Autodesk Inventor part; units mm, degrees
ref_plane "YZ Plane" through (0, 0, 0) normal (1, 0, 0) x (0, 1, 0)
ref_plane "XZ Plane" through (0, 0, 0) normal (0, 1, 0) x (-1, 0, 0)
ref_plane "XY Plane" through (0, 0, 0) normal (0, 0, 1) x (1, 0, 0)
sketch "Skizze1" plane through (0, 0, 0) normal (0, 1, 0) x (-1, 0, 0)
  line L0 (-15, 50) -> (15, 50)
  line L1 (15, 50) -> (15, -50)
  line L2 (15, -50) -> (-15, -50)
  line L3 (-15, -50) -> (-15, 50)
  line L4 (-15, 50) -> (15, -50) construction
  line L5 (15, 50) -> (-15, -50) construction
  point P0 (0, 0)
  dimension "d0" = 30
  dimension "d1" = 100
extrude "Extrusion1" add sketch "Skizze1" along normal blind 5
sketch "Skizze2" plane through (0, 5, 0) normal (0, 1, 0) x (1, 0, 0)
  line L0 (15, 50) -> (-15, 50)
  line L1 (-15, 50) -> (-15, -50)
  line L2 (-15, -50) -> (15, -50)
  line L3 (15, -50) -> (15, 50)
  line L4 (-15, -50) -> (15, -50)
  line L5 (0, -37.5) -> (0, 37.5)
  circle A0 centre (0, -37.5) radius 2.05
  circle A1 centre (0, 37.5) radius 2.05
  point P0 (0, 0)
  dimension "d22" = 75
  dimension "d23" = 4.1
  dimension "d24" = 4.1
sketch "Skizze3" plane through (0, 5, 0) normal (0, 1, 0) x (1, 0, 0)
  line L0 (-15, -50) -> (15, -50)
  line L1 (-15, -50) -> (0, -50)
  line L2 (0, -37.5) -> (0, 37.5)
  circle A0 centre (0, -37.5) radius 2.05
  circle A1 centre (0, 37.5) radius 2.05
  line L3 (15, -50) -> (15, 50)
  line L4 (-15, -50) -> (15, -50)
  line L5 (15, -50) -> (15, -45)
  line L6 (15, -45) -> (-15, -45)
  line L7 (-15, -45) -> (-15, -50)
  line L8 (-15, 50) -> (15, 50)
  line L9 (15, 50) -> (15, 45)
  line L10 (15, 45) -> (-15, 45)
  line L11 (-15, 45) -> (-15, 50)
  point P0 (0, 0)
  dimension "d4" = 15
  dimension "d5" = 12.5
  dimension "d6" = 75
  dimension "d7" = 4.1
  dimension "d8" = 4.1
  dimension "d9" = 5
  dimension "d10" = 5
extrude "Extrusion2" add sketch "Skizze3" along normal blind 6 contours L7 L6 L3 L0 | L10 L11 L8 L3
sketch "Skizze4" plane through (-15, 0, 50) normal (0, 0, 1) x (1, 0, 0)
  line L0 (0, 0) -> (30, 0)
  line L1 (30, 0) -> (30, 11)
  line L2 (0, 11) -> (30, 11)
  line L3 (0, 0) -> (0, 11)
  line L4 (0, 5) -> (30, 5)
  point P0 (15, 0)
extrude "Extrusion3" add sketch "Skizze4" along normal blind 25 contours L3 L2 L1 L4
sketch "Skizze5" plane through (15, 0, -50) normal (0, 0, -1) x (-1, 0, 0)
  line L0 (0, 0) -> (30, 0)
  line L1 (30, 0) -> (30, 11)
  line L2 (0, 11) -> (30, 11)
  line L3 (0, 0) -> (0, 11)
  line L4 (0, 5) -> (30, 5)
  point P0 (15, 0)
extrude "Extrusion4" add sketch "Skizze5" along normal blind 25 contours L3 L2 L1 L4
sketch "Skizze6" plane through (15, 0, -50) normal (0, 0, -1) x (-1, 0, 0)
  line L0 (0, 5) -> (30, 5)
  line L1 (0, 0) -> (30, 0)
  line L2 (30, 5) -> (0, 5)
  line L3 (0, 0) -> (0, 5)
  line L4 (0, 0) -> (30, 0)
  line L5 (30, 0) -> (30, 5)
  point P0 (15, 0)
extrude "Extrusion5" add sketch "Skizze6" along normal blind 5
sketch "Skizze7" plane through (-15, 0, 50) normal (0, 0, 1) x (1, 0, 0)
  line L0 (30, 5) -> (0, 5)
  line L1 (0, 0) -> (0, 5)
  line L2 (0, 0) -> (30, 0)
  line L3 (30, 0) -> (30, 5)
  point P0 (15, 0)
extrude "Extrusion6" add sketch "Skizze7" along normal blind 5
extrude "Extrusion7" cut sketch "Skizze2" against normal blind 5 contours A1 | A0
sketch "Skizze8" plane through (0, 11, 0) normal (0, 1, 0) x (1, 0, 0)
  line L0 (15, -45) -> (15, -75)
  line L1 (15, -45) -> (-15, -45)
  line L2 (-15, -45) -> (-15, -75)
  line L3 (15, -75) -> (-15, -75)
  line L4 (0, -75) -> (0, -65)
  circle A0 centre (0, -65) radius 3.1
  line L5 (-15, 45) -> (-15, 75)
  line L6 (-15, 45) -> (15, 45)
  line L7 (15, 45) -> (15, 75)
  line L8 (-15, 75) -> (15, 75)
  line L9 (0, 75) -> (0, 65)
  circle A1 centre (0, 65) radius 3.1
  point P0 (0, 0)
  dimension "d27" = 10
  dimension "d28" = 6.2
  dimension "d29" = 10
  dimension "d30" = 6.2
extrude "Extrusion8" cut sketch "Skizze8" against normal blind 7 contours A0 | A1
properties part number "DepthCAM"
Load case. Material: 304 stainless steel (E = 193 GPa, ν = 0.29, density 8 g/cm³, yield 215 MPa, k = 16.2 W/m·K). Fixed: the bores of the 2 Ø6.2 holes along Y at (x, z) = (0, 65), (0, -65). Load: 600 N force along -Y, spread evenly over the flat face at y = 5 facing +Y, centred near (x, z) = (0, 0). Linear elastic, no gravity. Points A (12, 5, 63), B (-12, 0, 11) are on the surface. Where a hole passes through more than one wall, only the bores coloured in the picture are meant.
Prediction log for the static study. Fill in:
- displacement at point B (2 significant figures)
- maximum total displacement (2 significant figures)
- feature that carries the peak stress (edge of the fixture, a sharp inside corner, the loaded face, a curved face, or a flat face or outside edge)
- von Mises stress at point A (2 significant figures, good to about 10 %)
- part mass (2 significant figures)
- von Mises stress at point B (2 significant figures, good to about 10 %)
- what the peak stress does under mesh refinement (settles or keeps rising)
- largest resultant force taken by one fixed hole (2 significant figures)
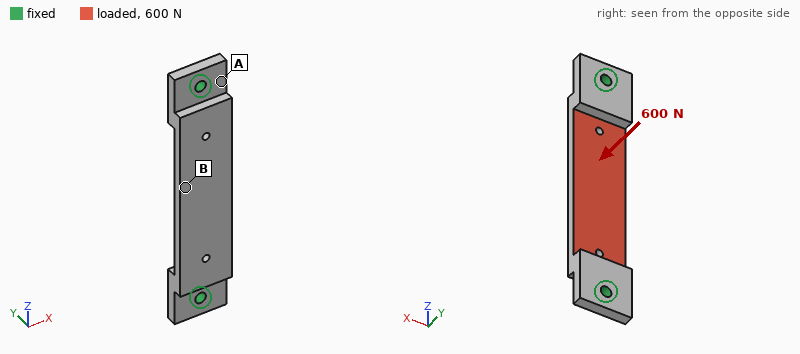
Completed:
35 µm
38 µm
edge of the fixture
8.1 MPa
210 g
27 MPa
keeps rising
950 N
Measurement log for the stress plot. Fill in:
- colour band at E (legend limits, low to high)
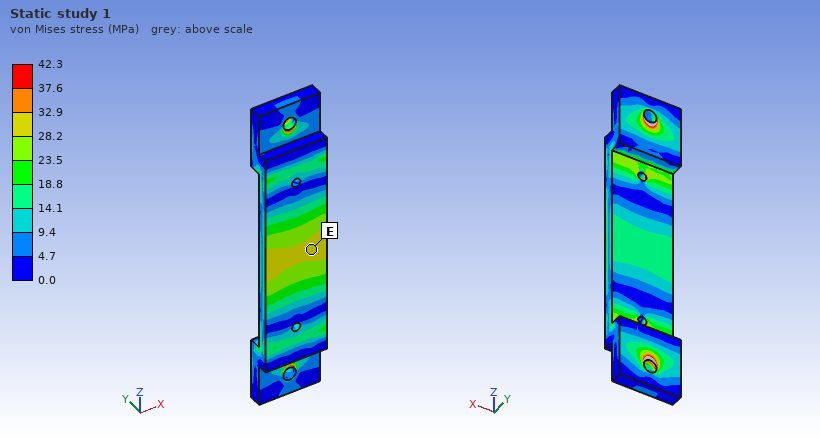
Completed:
28.2 to 32.9 MPa
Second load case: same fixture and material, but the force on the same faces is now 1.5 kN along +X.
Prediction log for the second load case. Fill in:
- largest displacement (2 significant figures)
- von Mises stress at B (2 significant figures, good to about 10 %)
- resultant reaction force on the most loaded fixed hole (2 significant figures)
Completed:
17 µm
22 MPa
750 N
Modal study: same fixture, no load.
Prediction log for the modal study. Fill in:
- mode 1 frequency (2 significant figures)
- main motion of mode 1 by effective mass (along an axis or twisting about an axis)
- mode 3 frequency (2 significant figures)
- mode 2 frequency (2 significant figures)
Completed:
2200 Hz
along Y
4400 Hz
4200 Hz
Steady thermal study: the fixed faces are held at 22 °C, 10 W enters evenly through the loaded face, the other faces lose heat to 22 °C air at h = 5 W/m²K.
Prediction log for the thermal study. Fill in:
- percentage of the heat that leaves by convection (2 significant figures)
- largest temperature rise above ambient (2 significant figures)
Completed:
15 %
73 K
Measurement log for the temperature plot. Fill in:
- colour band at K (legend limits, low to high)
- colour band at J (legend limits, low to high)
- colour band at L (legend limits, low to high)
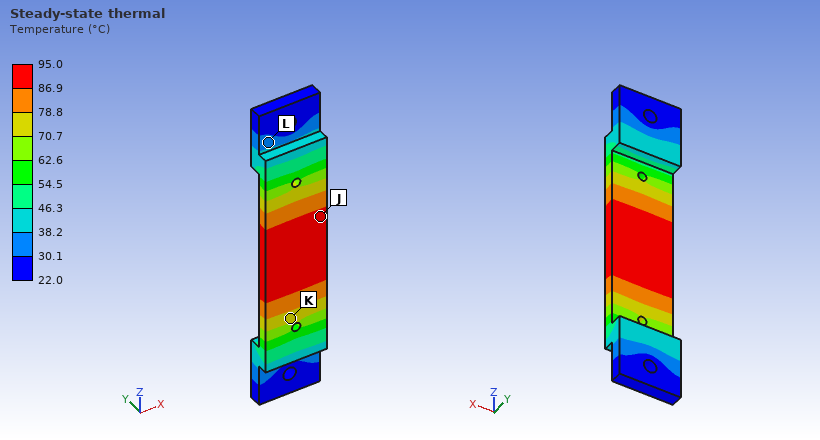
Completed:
70.7 to 78.8 °C
86.9 to 95.0 °C
30.1 to 38.2 °C
